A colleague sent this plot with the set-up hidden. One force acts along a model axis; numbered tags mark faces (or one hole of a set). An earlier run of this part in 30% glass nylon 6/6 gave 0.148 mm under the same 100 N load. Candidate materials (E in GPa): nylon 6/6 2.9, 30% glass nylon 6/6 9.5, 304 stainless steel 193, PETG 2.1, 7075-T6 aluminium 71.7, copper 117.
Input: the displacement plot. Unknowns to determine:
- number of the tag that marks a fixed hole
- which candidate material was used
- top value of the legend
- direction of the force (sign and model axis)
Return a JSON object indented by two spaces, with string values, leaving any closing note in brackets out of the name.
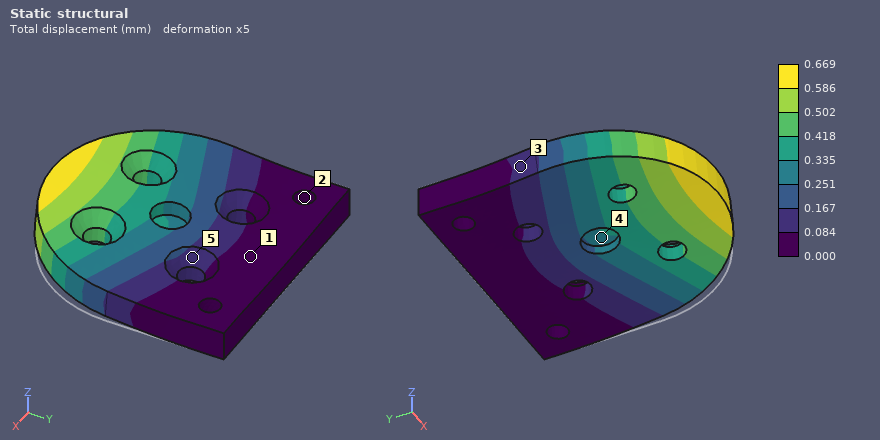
{
  "number of the tag that marks a fixed hole": "2",
  "which candidate material was used": "PETG",
  "top value of the legend": "0.669 mm",
  "direction of the force": "+Z"
}
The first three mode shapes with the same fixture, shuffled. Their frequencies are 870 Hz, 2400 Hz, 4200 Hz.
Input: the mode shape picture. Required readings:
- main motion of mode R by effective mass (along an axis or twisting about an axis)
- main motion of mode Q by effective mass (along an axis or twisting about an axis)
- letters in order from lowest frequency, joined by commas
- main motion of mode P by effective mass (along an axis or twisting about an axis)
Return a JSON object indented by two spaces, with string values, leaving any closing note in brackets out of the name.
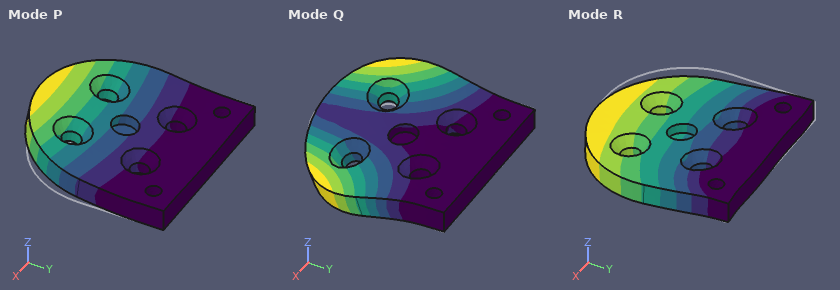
{
  "main motion of mode R by effective mass": "along X",
  "main motion of mode Q by effective mass": "twisting about Y",
  "letters in order from lowest frequency, joined by commas": "P, Q, R",
  "main motion of mode P by effective mass": "along Z"
}
